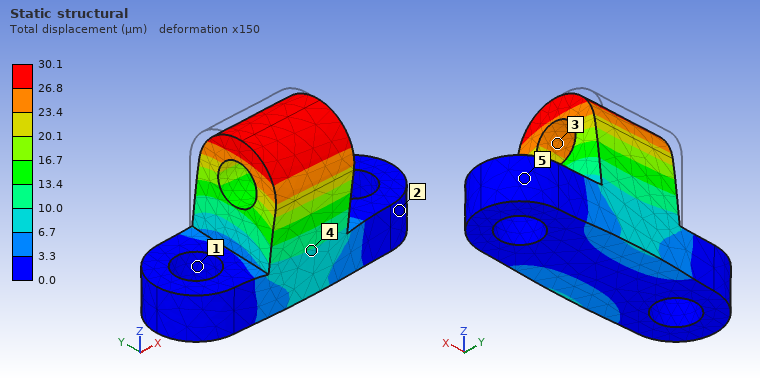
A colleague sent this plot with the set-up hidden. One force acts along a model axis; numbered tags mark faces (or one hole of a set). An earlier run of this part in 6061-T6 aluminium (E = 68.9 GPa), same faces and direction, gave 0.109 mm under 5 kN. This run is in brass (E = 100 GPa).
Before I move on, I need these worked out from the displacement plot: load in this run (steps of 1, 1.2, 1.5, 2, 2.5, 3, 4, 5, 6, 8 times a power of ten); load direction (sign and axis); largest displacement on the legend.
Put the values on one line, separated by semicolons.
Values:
2 kN; -Y; 30.1 µm
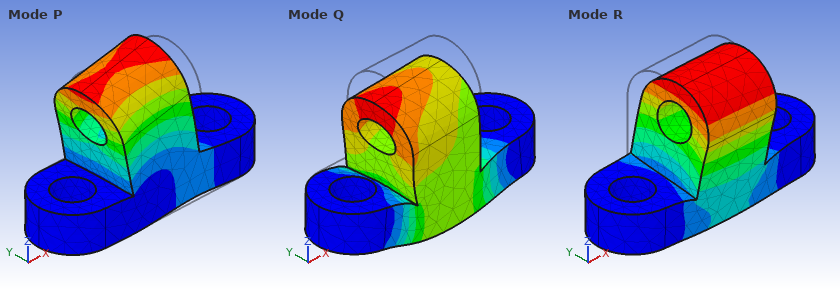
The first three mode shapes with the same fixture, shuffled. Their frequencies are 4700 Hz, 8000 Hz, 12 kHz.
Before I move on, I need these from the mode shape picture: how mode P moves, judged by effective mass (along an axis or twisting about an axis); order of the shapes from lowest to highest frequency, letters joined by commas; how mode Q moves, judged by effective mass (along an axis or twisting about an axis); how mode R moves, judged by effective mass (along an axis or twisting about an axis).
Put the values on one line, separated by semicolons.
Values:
along X; R, P, Q; along Z; along Y
